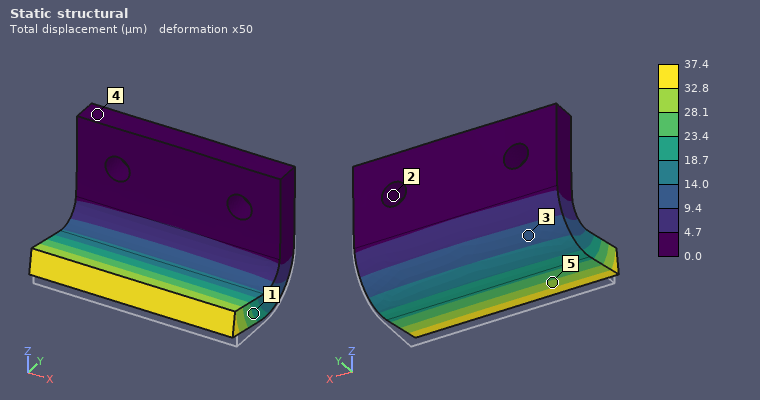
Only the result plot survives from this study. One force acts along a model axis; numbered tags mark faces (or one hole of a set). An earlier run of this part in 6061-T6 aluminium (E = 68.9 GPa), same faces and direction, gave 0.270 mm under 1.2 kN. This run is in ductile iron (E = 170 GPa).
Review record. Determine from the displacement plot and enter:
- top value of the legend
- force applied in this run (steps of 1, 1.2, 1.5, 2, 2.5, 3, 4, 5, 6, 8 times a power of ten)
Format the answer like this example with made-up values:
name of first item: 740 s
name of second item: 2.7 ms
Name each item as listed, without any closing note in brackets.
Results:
top value of the legend: 37.4 µm
force applied in this run: 400 N
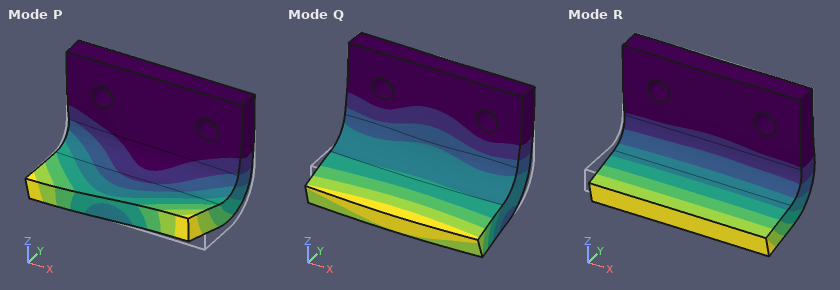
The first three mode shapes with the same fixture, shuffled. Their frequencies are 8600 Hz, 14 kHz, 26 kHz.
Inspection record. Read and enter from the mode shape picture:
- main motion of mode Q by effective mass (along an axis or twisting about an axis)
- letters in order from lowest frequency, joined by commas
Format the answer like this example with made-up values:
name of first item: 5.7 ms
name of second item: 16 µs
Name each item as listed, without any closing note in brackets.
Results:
main motion of mode Q by effective mass: along Y
letters in order from lowest frequency, joined by commas: R, P, Q
